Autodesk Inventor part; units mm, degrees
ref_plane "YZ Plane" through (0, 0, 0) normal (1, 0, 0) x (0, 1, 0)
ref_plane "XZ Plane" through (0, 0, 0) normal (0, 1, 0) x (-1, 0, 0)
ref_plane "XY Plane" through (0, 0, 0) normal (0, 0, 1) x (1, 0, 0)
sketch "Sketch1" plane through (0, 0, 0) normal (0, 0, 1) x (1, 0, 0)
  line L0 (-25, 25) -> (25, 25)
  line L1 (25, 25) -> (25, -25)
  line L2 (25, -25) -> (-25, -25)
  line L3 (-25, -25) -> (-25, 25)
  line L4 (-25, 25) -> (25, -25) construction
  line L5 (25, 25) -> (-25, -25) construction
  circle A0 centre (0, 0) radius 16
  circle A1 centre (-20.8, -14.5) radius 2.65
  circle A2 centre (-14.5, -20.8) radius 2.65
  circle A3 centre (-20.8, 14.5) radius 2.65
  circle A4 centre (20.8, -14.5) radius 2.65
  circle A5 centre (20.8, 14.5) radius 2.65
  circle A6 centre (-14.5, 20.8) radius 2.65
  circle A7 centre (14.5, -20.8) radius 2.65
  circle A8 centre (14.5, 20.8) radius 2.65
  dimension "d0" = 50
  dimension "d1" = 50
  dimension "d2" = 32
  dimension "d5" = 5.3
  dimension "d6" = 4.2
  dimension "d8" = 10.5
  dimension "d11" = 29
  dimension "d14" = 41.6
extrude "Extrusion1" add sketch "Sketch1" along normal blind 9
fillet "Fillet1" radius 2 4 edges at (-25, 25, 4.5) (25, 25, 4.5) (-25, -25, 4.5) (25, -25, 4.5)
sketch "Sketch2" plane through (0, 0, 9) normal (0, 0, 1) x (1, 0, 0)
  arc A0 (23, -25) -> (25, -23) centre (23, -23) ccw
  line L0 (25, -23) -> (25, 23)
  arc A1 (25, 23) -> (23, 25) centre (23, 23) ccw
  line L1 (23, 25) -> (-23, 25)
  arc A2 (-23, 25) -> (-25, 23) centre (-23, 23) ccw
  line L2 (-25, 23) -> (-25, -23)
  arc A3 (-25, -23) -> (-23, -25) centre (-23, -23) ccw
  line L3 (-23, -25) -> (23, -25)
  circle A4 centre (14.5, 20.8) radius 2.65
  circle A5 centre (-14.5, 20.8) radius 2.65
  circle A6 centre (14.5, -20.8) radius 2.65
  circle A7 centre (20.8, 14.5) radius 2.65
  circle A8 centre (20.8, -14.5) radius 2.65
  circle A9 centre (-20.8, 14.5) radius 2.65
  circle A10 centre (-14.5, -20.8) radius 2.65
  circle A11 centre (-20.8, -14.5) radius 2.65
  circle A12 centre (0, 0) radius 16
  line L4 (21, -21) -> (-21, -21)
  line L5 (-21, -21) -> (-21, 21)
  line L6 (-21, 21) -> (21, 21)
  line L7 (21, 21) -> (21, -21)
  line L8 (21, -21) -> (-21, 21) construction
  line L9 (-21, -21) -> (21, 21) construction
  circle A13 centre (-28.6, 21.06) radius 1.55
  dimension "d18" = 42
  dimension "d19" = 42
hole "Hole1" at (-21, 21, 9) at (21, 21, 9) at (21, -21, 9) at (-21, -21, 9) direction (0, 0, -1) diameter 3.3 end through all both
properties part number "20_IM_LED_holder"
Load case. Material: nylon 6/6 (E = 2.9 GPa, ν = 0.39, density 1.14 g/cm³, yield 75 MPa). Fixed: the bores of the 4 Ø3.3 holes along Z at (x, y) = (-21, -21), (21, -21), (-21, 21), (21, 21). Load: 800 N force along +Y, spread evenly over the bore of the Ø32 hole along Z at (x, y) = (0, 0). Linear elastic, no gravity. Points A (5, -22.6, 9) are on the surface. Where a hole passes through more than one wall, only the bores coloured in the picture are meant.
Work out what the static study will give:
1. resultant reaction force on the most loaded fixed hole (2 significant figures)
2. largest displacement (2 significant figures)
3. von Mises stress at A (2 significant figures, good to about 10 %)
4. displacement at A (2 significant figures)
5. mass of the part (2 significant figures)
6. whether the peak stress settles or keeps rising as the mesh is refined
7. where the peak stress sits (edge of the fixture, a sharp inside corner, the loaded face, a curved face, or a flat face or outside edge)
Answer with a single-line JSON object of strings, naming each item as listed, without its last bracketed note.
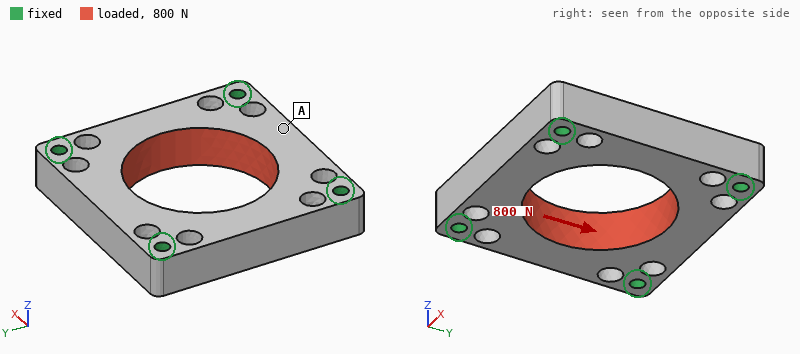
{"resultant reaction force on the most loaded fixed hole": "210 N", "largest displacement": "45 µm", "von Mises stress at A": "1.7 MPa", "displacement at A": "40 µm", "mass of the part": "15 g", "whether the peak stress settles or keeps rising as the mesh is refined": "keeps rising", "where the peak stress sits": "edge of the fixture"}
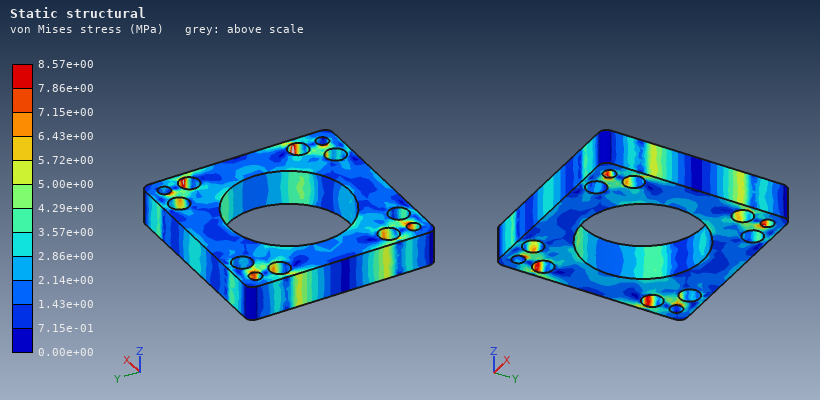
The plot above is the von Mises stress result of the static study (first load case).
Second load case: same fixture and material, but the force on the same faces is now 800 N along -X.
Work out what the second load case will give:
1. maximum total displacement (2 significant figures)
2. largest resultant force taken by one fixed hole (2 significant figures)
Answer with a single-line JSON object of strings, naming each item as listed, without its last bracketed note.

{"maximum total displacement": "45 µm", "largest resultant force taken by one fixed hole": "210 N"}
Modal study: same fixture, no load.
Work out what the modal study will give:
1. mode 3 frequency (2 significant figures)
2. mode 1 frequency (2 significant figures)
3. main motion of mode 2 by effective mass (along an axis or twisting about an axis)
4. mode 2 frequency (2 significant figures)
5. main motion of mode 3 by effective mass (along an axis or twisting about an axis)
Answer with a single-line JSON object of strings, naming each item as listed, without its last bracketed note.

{"mode 3 frequency": "5900 Hz", "mode 1 frequency": "4600 Hz", "main motion of mode 2 by effective mass": "along Z", "mode 2 frequency": "5200 Hz", "main motion of mode 3 by effective mass": "twisting about X"}
